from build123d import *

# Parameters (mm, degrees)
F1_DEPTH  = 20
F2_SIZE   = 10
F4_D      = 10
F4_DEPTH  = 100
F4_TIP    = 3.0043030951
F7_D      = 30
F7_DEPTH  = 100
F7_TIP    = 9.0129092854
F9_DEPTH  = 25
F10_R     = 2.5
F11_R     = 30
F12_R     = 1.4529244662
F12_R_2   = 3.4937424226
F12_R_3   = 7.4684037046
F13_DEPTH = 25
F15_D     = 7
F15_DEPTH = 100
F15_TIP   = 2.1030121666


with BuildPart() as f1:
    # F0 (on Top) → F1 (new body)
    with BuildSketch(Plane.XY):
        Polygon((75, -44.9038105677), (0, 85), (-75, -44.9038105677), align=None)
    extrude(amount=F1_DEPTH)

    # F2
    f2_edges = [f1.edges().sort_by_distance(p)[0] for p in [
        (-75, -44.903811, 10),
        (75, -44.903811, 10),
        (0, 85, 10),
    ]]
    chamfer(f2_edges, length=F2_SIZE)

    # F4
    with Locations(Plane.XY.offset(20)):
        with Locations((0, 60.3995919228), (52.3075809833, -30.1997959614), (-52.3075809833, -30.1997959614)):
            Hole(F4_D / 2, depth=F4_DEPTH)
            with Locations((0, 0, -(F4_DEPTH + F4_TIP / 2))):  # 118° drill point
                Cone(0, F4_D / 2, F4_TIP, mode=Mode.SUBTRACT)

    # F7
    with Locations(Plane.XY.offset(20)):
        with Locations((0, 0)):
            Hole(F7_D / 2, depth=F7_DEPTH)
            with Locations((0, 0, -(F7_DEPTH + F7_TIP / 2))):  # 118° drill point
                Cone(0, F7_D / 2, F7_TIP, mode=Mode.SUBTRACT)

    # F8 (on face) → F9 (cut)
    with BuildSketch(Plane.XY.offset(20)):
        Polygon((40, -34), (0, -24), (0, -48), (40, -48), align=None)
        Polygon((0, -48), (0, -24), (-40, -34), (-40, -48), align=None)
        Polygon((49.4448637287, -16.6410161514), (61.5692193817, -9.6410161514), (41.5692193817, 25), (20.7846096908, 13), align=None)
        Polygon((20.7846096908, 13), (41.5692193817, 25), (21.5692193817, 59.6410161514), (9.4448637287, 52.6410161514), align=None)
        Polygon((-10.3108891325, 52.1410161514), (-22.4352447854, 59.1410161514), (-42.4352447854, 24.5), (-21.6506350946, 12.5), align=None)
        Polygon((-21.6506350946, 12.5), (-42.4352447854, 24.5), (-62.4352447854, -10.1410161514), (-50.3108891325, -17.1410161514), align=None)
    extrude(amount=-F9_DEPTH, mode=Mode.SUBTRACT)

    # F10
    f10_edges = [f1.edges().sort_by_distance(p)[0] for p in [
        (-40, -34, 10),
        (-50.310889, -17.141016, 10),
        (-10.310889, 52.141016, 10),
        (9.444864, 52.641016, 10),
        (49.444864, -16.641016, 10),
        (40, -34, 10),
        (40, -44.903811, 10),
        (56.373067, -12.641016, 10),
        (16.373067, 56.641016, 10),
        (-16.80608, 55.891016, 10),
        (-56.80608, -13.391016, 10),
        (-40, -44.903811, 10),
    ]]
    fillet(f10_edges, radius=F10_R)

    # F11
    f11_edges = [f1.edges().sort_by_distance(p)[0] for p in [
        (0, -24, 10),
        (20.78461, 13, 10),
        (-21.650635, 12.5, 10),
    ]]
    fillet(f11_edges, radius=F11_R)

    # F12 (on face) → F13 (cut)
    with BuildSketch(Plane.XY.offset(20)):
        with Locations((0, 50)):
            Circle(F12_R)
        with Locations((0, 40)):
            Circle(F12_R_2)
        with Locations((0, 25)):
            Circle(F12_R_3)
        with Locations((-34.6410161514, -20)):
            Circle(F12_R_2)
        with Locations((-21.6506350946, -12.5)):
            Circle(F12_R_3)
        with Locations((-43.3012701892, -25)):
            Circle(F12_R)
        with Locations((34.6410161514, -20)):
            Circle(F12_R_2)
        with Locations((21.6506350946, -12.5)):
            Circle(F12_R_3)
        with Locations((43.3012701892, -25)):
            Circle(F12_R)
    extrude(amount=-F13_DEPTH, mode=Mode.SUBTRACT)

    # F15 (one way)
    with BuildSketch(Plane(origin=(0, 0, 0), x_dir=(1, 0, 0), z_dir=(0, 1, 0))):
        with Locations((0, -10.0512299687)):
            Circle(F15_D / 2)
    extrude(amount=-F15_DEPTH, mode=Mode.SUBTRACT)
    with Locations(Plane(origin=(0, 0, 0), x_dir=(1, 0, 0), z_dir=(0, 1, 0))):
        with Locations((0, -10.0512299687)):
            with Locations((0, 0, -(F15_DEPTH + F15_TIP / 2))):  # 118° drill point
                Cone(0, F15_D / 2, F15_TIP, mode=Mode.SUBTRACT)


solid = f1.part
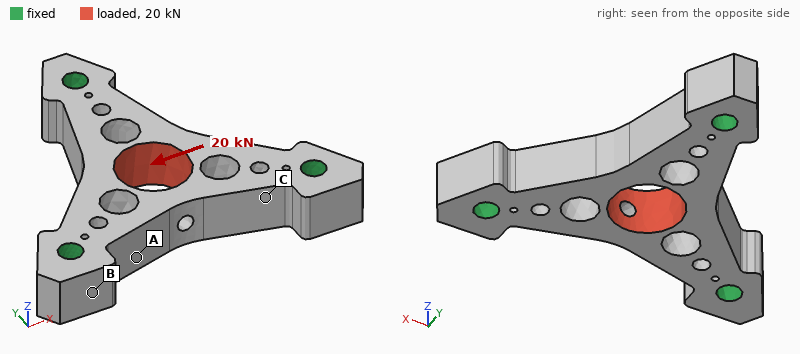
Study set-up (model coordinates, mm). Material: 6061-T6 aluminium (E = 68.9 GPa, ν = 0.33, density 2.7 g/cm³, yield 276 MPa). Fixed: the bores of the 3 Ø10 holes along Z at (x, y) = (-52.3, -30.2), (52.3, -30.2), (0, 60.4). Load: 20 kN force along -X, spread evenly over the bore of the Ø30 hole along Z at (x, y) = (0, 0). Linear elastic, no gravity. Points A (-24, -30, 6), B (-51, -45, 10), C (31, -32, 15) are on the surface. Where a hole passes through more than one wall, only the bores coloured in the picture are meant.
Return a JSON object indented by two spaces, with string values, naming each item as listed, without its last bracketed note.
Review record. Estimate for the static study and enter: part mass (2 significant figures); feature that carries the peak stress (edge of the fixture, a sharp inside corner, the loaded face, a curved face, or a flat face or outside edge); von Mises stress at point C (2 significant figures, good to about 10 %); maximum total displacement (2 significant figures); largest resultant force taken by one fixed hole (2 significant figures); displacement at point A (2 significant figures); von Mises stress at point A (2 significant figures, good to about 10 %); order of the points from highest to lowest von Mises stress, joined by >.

{
  "part mass": "250 g",
  "feature that carries the peak stress": "a curved face",
  "von Mises stress at point C": "25 MPa",
  "maximum total displacement": "46 µm",
  "largest resultant force taken by one fixed hole": "10 kN",
  "displacement at point A": "10 µm",
  "von Mises stress at point A": "32 MPa",
  "order of the points from highest to lowest von Mises stress, joined by >": "A > C > B"
}
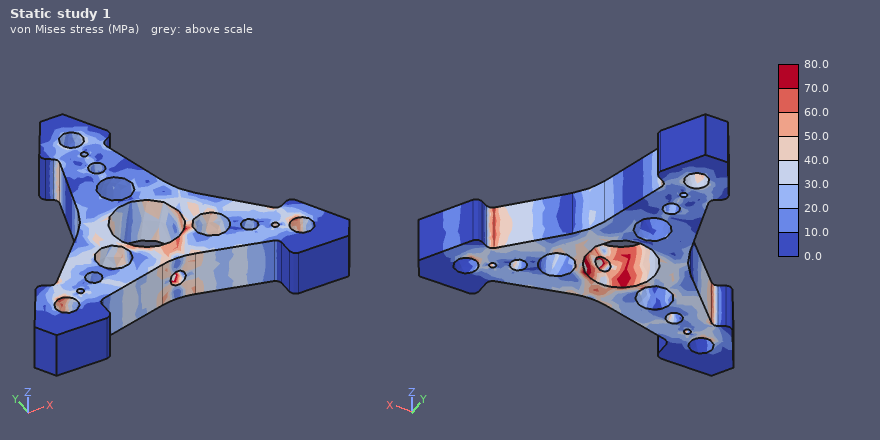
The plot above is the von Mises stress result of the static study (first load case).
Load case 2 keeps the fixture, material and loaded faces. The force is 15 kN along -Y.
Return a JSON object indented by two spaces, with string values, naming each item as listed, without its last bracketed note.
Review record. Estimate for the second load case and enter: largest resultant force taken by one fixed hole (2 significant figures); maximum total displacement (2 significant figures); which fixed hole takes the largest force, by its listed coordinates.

{
  "largest resultant force taken by one fixed hole": "8.7 kN",
  "maximum total displacement": "36 µm",
  "which fixed hole takes the largest force, by its listed coordinates": "(0, 60.4)"
}
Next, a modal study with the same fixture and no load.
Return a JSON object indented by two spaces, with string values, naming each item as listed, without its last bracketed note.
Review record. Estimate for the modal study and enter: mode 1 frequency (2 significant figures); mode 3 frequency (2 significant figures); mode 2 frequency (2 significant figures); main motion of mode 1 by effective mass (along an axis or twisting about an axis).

{
  "mode 1 frequency": "7500 Hz",
  "mode 3 frequency": "11 kHz",
  "mode 2 frequency": "11 kHz",
  "main motion of mode 1 by effective mass": "along Z"
}
